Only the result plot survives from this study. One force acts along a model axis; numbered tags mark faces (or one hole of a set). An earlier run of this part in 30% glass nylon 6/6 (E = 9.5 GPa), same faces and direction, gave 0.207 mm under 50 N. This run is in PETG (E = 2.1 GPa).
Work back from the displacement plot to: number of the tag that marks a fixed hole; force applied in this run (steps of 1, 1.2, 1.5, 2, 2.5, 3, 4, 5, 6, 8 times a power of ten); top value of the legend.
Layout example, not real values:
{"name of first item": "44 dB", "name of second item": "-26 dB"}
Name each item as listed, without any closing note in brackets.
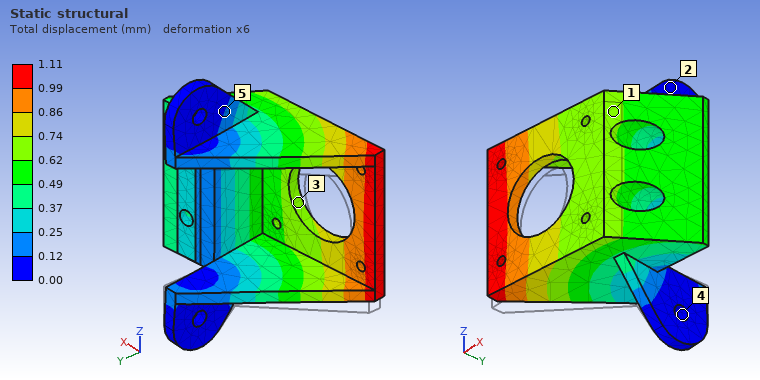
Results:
{"number of the tag that marks a fixed hole": "4", "force applied in this run": "60 N", "top value of the legend": "1.11 mm"}
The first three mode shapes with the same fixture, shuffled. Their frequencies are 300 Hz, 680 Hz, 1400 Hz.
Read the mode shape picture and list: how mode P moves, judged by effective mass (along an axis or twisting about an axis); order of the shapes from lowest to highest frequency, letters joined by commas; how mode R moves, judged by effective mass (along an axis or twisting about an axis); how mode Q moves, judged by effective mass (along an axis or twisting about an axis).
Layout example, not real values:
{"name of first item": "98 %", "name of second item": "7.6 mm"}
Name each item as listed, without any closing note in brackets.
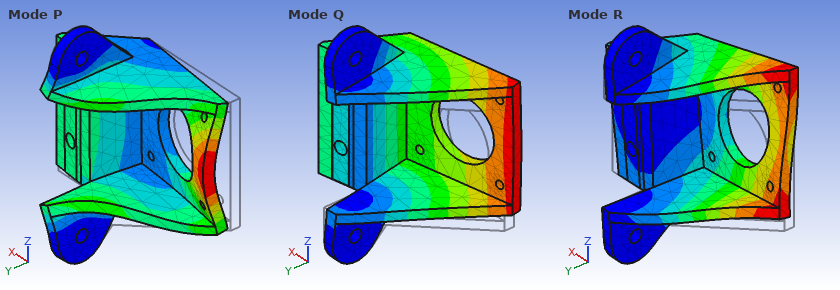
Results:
{"how mode P moves, judged by effective mass": "along X", "order of the shapes from lowest to highest frequency, letters joined by commas": "Q, R, P", "how mode R moves, judged by effective mass": "along Z", "how mode Q moves, judged by effective mass": "along X"}
